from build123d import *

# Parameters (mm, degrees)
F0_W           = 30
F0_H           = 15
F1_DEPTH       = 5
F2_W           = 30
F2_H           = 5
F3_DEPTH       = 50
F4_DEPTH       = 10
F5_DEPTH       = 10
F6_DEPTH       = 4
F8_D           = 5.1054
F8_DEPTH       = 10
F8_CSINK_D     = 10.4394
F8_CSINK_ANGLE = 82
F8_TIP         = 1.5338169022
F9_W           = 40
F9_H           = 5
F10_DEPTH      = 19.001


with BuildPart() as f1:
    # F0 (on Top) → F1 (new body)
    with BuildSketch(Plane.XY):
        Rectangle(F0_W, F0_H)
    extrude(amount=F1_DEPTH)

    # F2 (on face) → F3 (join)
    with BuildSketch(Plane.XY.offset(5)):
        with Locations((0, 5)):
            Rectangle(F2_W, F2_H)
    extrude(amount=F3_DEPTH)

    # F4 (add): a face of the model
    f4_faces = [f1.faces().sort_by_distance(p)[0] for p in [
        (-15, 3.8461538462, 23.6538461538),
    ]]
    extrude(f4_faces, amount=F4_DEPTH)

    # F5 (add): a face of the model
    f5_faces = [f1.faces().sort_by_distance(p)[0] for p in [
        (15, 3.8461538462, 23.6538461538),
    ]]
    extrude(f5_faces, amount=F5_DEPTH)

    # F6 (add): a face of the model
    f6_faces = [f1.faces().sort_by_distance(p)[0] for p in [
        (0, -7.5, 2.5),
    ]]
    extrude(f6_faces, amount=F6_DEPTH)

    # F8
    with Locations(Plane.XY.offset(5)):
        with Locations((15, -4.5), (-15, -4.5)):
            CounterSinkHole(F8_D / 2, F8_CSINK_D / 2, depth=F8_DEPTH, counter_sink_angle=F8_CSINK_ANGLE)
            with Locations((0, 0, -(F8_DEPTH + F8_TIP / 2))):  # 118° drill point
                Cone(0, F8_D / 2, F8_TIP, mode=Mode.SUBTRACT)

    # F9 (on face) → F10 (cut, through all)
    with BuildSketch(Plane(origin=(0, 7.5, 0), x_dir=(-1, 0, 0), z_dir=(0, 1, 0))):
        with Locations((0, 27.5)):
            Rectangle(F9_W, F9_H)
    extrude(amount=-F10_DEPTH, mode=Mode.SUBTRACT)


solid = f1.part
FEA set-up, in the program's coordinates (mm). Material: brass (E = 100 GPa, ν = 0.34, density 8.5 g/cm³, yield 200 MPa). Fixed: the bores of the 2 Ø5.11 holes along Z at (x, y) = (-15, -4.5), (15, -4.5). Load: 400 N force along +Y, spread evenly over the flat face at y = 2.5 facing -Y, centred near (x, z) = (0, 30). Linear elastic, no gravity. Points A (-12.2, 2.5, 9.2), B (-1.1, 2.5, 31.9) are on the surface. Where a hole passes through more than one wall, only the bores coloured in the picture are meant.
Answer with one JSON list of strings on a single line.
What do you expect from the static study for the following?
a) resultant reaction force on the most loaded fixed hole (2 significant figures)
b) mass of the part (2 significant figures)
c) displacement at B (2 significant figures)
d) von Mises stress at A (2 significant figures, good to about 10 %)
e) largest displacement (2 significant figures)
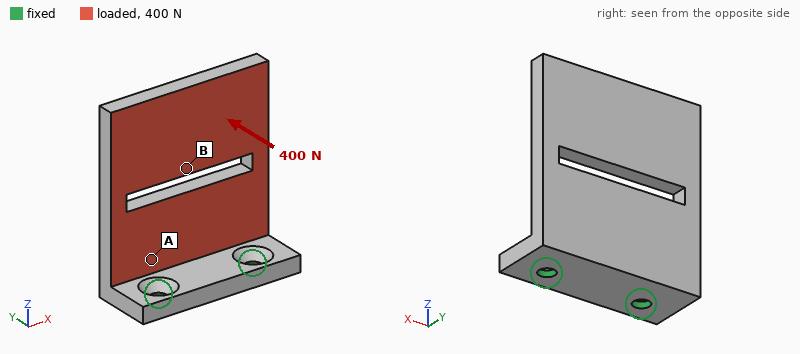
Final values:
["220 N", "130 g", "0.21 mm", "35 MPa", "0.47 mm"]
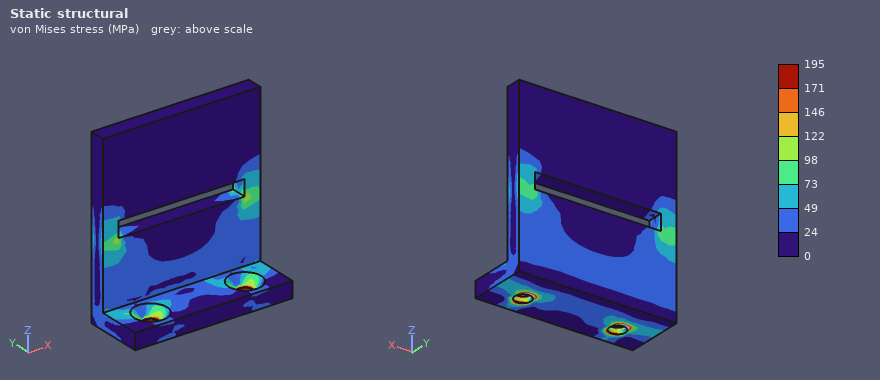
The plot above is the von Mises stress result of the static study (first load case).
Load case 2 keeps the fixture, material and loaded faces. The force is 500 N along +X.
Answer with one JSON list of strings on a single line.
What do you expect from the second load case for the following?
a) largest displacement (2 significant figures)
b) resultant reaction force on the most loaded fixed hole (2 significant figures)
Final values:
["50 µm", "530 N"]
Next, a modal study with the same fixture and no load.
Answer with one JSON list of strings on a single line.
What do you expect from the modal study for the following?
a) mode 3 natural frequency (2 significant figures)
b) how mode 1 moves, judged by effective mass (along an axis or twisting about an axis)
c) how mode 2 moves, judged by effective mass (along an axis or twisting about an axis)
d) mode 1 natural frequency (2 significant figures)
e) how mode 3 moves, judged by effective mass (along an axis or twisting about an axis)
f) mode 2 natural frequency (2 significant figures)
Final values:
["2500 Hz", "along Y", "along X", "580 Hz", "along X", "1800 Hz"]
